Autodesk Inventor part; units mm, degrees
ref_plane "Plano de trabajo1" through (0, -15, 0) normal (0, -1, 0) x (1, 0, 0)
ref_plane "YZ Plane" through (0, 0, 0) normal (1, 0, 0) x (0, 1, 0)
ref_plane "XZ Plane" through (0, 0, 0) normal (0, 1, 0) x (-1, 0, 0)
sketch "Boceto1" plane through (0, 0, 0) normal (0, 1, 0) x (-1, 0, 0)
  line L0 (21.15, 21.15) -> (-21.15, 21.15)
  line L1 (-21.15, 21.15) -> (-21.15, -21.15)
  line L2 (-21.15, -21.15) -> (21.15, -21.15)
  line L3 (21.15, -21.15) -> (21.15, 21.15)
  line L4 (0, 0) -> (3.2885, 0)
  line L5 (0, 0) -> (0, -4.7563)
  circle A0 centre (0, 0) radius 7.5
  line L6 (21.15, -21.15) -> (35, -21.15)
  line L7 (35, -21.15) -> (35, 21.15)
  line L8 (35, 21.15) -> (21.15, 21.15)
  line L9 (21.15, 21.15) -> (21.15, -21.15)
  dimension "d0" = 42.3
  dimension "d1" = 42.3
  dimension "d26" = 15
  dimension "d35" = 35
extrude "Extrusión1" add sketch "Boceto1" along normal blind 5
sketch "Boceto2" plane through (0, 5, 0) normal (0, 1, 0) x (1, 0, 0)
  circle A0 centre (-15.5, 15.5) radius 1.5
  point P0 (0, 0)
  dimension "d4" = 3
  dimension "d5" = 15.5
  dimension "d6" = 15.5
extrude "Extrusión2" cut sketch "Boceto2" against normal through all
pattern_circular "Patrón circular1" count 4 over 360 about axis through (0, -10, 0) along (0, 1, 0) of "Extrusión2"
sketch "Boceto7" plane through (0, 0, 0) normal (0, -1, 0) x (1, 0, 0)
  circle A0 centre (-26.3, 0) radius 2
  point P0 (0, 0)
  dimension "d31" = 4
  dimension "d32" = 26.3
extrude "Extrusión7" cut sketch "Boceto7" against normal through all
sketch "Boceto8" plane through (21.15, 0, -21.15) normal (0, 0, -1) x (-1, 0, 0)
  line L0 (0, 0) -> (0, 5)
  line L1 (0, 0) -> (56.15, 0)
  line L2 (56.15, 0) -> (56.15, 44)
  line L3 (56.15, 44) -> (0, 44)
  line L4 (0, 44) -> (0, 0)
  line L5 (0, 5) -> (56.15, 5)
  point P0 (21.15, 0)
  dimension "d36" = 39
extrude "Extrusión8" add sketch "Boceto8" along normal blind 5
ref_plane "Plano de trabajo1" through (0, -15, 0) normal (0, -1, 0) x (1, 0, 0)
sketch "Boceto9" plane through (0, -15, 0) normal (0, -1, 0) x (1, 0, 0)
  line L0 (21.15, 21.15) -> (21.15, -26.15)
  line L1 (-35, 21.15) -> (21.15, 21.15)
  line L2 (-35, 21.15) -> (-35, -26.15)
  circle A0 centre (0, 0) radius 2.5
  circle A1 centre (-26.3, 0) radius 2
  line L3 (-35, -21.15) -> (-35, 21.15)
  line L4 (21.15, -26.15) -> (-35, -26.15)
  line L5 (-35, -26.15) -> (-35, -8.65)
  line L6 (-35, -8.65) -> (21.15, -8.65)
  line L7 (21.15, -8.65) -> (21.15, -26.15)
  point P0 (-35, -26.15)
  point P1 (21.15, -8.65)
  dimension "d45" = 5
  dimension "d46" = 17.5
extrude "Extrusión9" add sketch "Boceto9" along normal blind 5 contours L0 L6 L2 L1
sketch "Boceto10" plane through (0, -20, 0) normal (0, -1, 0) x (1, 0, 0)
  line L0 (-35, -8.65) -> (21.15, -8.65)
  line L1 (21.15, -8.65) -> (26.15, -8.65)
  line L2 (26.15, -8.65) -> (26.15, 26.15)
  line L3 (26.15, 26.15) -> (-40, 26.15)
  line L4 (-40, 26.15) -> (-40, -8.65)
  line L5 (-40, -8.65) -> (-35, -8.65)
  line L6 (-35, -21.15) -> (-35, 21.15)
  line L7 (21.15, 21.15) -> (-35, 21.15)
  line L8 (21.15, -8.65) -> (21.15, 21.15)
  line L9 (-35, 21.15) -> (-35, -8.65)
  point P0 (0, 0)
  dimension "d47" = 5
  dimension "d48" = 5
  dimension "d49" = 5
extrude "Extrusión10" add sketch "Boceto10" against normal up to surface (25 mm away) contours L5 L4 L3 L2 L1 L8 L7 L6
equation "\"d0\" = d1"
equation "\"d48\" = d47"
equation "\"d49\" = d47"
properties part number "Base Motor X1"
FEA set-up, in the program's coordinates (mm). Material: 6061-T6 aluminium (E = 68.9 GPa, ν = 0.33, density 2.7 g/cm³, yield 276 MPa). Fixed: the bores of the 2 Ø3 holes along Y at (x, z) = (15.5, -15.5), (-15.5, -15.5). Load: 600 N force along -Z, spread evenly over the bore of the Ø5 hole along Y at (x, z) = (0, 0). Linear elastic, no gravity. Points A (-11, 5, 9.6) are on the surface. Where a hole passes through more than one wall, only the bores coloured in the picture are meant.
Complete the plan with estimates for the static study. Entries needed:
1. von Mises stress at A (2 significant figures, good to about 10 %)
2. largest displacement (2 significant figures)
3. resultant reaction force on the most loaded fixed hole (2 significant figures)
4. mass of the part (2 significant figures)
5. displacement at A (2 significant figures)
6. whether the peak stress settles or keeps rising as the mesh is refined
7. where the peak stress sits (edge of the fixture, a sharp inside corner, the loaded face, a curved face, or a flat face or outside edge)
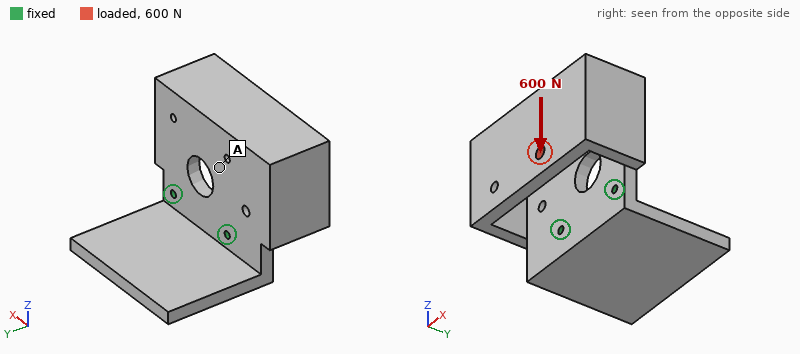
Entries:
12 MPa
0.26 mm
310 N
130 g
0.11 mm
keeps rising
edge of the fixture
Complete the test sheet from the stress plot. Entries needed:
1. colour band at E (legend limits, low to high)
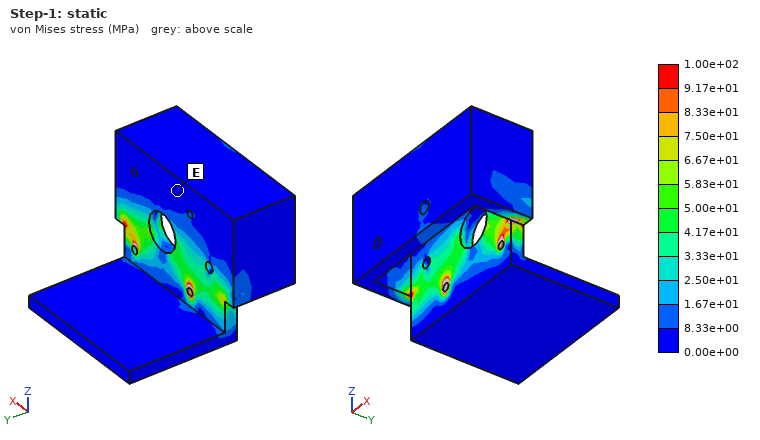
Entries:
0.00e+00 to 8.33e+00 MPa
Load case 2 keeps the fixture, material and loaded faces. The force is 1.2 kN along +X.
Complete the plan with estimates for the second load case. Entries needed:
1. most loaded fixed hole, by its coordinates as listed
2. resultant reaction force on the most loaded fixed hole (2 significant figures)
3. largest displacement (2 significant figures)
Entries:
(-15.5, -15.5)
1.1 kN
0.21 mm
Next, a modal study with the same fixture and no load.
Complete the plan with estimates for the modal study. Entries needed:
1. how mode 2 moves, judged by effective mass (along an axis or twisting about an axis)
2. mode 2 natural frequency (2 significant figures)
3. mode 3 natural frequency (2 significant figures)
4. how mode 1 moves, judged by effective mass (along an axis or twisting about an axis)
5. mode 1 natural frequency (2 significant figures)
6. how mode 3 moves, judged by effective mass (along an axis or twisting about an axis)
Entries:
along Z
1700 Hz
2000 Hz
along Y
890 Hz
along X
